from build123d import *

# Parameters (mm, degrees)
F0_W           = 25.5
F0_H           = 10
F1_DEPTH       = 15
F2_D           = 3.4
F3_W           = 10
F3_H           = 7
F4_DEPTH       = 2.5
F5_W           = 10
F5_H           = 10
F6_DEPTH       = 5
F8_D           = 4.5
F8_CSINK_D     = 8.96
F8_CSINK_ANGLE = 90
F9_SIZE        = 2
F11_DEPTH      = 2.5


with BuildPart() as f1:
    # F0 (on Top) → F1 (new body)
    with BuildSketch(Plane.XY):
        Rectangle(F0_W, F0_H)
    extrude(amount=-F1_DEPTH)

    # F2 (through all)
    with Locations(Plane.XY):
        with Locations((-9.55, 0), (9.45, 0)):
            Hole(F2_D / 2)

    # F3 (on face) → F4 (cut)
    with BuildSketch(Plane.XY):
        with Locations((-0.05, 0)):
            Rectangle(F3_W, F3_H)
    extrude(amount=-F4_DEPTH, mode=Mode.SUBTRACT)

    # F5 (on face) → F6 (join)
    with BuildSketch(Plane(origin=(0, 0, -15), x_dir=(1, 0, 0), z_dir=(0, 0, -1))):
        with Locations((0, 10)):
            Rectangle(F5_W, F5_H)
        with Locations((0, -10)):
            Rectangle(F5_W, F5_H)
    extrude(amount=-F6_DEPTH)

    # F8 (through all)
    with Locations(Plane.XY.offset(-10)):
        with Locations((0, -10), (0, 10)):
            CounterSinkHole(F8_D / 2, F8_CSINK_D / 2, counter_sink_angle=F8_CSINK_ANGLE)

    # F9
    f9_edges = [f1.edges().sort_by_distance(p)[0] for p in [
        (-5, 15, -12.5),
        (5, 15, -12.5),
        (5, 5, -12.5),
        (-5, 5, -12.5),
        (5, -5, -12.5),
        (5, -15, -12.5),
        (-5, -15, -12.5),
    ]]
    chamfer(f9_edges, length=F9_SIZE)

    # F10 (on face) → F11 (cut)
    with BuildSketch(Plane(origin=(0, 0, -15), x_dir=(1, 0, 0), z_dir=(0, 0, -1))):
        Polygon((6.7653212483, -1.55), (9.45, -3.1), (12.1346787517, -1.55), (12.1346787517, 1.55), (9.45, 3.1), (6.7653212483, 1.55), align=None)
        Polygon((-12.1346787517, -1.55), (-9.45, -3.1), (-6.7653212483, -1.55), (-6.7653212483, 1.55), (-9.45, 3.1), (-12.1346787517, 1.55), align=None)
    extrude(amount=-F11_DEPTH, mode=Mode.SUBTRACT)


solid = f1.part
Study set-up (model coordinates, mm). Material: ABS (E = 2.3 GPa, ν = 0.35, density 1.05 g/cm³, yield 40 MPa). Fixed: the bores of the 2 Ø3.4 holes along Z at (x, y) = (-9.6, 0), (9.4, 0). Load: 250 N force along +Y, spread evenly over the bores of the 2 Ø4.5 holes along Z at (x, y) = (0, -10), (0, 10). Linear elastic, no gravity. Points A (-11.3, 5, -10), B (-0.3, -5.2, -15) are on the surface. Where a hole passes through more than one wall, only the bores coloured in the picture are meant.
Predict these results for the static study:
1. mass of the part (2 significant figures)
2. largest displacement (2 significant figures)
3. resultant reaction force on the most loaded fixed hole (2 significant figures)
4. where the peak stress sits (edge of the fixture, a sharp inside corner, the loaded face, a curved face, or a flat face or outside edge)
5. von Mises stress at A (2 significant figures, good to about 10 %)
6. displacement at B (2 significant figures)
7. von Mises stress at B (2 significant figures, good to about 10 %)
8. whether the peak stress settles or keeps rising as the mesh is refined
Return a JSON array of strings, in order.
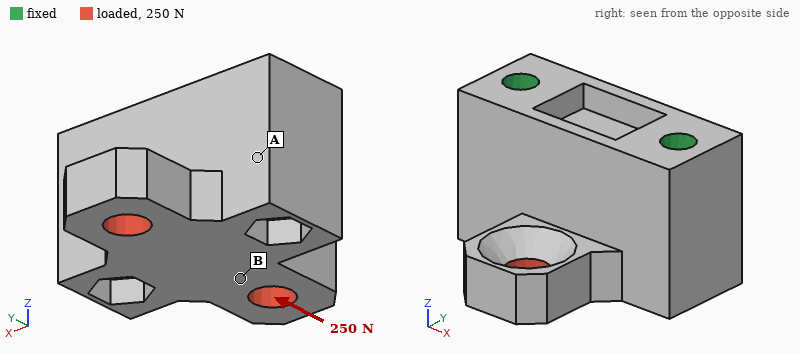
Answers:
["4.2 g", "0.10 mm", "130 N", "edge of the fixture", "1.5 MPa", "0.039 mm", "3.7 MPa", "keeps rising"]
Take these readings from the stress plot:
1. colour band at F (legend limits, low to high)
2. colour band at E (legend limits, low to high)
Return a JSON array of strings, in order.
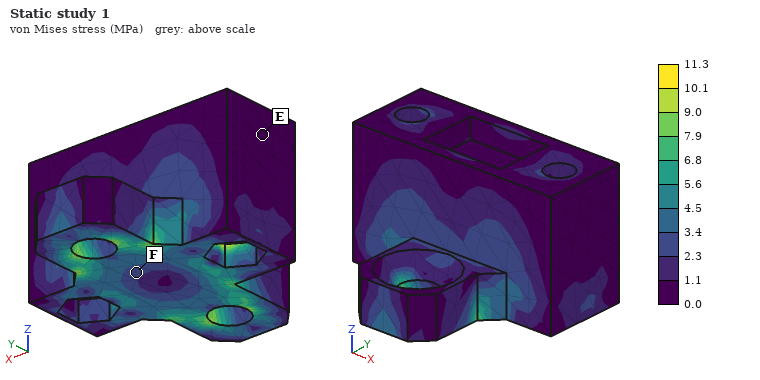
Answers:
["2.3 to 3.4 MPa", "0.0 to 1.1 MPa"]
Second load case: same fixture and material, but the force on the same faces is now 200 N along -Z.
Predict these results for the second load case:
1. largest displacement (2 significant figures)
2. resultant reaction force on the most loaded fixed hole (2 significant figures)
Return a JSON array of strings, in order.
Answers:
["0.16 mm", "110 N"]
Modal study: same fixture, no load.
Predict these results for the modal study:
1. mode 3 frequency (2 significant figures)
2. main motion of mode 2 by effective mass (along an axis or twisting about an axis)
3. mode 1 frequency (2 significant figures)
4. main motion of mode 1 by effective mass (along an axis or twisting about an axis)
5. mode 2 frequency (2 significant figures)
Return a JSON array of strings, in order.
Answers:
["10 kHz", "along Z", "6700 Hz", "twisting about X", "7800 Hz"]
